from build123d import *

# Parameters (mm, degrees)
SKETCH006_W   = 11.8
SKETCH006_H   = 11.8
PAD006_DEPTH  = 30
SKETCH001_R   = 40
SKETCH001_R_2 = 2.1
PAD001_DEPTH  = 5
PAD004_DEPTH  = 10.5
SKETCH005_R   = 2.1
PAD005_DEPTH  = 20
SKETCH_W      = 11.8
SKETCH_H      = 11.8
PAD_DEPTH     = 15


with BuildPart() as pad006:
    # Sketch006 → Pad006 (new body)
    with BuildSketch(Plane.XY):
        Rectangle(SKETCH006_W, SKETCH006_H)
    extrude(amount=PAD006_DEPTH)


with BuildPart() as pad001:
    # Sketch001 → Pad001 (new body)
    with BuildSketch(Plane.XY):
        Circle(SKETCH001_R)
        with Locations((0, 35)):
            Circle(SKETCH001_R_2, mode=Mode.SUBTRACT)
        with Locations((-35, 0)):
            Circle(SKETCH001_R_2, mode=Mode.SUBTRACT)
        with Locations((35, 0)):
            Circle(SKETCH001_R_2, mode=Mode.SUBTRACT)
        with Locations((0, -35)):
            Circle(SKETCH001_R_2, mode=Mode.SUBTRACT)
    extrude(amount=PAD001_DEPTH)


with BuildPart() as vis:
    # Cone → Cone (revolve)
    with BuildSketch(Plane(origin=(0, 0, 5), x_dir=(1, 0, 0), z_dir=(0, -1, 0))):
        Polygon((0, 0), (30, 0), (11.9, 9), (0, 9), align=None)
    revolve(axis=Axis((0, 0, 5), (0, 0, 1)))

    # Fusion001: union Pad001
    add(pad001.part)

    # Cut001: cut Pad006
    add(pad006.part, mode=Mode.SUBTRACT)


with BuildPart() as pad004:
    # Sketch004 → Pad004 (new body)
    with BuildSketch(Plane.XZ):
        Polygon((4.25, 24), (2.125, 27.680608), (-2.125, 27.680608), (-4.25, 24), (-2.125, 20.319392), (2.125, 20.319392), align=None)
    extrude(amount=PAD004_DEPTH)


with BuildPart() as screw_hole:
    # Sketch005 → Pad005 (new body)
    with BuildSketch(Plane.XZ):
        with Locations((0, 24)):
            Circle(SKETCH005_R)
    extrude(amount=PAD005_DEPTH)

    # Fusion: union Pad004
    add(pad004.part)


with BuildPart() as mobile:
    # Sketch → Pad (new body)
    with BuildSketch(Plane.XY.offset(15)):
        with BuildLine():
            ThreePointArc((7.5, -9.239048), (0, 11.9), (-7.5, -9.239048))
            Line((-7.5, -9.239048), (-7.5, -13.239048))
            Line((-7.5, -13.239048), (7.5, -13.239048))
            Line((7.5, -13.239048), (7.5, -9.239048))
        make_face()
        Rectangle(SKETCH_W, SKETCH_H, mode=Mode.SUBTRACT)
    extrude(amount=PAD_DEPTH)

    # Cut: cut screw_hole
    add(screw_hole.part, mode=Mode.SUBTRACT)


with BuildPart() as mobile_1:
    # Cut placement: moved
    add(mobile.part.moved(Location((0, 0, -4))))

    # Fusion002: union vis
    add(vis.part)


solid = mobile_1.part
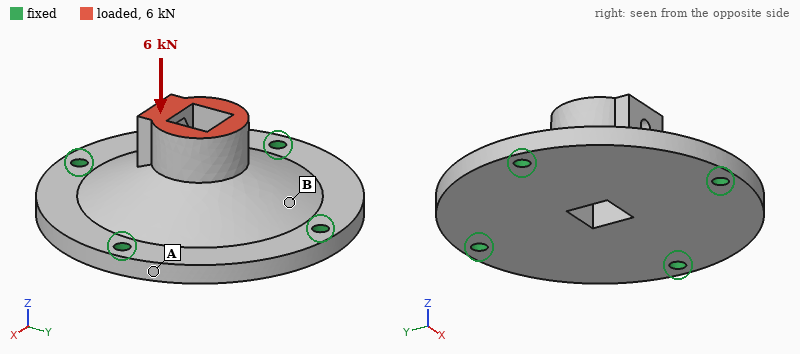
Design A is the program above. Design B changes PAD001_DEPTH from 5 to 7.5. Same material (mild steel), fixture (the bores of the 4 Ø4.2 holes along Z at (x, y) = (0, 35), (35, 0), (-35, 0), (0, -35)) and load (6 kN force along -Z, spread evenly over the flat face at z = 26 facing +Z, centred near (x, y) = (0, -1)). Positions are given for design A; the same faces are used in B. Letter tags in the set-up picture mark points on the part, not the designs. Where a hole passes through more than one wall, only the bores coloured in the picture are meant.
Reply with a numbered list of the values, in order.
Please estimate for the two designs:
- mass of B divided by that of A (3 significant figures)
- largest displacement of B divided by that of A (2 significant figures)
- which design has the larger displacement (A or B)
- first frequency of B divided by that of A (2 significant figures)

1. 1.16
2. 0.81
3. A
4. 1.2
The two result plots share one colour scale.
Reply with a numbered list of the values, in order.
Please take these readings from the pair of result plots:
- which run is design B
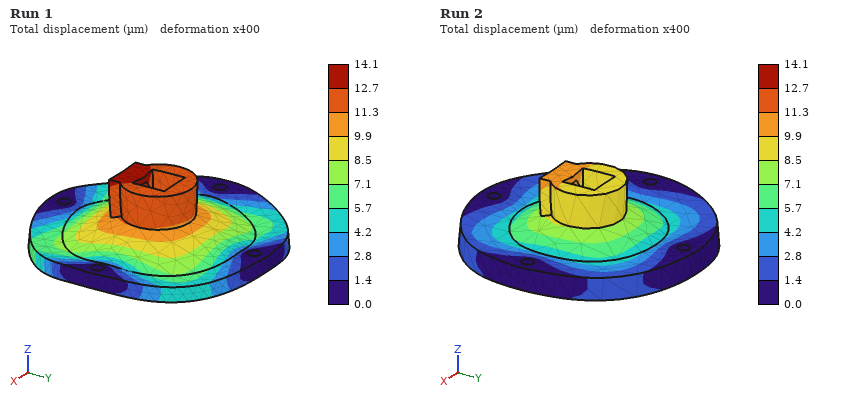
1. Run 2
